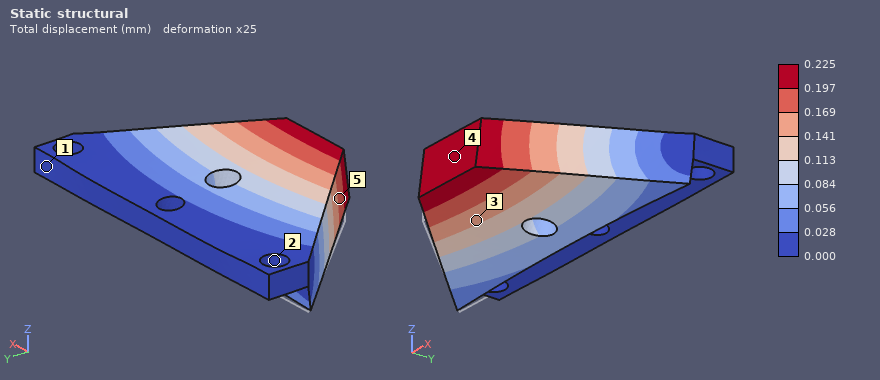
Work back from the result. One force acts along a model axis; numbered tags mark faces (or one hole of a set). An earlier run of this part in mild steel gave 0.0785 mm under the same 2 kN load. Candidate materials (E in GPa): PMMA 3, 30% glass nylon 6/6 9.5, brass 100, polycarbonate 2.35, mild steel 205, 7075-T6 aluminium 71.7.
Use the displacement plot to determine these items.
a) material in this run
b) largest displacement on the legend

7075-T6 aluminium
0.225 mm
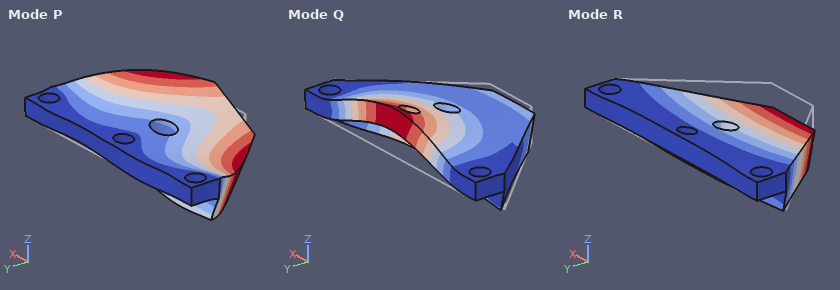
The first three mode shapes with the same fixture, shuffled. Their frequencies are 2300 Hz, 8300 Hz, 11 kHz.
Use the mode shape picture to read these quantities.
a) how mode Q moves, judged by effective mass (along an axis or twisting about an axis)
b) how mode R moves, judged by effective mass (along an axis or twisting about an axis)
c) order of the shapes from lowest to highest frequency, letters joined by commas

along Z
along Z
R, Q, P
